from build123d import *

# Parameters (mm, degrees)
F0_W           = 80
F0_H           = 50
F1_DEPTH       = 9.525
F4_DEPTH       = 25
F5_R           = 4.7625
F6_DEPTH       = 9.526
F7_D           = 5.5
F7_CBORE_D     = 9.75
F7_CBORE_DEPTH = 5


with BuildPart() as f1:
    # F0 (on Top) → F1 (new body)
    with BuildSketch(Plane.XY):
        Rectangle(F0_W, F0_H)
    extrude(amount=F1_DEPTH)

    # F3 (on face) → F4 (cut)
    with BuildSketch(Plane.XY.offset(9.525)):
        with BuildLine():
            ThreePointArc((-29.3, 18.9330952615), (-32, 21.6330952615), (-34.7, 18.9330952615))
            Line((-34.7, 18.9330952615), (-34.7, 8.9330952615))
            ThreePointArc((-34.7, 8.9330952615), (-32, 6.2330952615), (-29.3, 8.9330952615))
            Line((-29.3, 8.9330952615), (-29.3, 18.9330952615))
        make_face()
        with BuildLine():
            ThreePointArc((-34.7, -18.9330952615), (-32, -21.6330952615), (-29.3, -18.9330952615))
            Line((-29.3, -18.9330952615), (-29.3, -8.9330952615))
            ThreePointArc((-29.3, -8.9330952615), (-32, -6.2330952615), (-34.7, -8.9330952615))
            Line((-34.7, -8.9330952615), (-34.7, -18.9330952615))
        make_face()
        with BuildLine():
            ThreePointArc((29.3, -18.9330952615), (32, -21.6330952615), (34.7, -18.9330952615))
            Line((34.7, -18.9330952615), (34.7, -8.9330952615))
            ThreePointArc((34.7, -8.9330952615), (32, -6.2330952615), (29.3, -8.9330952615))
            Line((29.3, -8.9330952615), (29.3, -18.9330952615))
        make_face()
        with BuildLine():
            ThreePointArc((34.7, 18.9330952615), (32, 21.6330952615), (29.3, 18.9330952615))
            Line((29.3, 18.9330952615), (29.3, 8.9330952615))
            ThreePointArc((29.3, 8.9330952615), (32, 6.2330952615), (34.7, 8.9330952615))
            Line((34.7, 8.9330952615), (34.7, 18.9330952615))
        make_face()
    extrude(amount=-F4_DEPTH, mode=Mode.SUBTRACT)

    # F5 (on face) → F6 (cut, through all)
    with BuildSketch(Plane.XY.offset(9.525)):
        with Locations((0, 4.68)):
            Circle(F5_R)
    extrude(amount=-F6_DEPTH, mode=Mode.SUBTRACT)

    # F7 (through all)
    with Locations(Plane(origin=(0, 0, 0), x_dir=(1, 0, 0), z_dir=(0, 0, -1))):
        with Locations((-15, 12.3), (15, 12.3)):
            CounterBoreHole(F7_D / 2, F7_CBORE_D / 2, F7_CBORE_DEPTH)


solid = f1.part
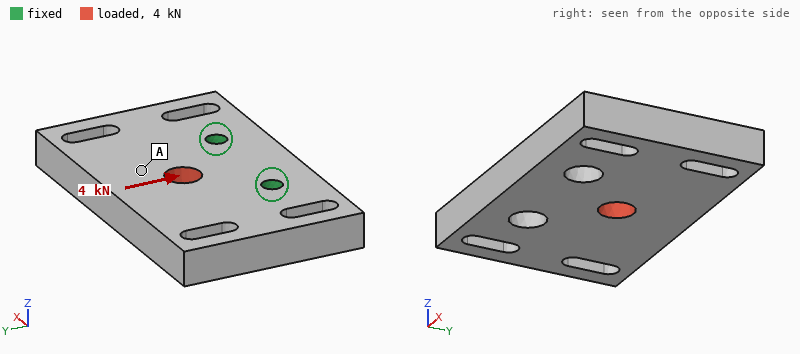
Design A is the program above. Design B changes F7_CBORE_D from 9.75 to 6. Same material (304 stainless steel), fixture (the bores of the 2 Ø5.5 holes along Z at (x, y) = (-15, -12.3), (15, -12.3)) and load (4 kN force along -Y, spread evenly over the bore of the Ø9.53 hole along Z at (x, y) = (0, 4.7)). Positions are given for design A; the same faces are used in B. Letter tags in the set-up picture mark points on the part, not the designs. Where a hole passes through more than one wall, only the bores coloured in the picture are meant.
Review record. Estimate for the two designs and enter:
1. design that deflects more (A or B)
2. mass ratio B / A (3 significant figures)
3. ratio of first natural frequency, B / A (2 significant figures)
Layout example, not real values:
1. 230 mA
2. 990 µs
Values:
1. A
2. 1.01
3. 1.1
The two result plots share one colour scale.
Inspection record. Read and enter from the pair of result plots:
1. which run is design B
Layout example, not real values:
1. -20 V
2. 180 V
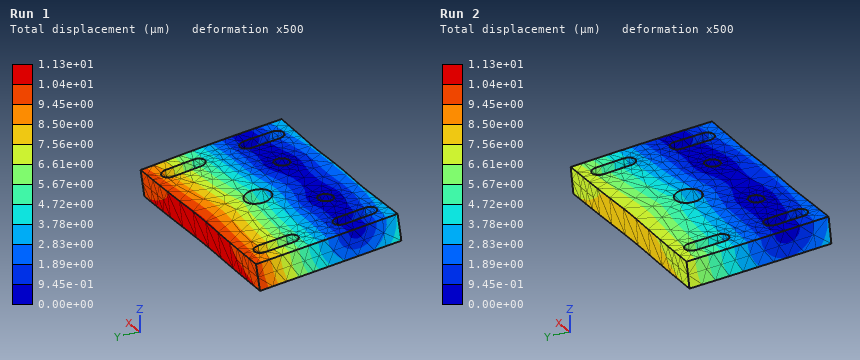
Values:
1. Run 2
